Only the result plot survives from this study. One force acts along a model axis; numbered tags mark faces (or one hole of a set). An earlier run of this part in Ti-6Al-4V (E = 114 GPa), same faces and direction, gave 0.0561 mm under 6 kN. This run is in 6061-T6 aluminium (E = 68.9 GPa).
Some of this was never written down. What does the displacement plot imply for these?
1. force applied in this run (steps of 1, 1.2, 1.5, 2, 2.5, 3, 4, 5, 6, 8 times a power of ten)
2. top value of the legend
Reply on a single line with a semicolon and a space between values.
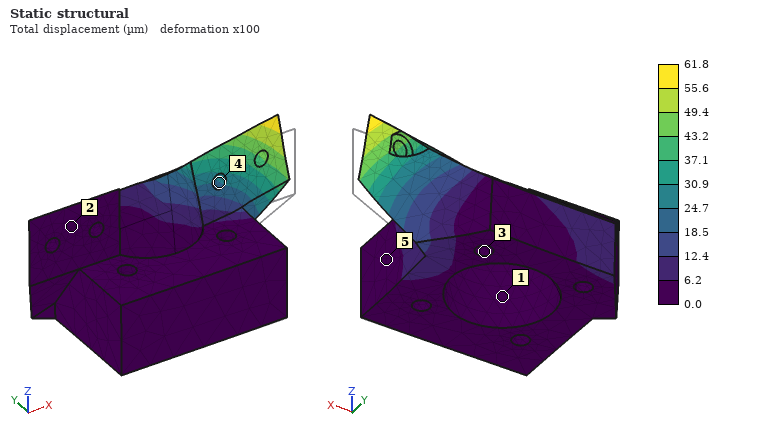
4 kN; 61.8 µm
